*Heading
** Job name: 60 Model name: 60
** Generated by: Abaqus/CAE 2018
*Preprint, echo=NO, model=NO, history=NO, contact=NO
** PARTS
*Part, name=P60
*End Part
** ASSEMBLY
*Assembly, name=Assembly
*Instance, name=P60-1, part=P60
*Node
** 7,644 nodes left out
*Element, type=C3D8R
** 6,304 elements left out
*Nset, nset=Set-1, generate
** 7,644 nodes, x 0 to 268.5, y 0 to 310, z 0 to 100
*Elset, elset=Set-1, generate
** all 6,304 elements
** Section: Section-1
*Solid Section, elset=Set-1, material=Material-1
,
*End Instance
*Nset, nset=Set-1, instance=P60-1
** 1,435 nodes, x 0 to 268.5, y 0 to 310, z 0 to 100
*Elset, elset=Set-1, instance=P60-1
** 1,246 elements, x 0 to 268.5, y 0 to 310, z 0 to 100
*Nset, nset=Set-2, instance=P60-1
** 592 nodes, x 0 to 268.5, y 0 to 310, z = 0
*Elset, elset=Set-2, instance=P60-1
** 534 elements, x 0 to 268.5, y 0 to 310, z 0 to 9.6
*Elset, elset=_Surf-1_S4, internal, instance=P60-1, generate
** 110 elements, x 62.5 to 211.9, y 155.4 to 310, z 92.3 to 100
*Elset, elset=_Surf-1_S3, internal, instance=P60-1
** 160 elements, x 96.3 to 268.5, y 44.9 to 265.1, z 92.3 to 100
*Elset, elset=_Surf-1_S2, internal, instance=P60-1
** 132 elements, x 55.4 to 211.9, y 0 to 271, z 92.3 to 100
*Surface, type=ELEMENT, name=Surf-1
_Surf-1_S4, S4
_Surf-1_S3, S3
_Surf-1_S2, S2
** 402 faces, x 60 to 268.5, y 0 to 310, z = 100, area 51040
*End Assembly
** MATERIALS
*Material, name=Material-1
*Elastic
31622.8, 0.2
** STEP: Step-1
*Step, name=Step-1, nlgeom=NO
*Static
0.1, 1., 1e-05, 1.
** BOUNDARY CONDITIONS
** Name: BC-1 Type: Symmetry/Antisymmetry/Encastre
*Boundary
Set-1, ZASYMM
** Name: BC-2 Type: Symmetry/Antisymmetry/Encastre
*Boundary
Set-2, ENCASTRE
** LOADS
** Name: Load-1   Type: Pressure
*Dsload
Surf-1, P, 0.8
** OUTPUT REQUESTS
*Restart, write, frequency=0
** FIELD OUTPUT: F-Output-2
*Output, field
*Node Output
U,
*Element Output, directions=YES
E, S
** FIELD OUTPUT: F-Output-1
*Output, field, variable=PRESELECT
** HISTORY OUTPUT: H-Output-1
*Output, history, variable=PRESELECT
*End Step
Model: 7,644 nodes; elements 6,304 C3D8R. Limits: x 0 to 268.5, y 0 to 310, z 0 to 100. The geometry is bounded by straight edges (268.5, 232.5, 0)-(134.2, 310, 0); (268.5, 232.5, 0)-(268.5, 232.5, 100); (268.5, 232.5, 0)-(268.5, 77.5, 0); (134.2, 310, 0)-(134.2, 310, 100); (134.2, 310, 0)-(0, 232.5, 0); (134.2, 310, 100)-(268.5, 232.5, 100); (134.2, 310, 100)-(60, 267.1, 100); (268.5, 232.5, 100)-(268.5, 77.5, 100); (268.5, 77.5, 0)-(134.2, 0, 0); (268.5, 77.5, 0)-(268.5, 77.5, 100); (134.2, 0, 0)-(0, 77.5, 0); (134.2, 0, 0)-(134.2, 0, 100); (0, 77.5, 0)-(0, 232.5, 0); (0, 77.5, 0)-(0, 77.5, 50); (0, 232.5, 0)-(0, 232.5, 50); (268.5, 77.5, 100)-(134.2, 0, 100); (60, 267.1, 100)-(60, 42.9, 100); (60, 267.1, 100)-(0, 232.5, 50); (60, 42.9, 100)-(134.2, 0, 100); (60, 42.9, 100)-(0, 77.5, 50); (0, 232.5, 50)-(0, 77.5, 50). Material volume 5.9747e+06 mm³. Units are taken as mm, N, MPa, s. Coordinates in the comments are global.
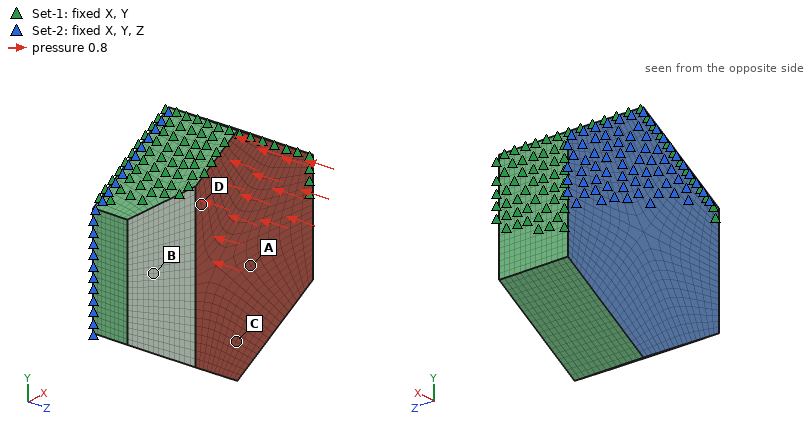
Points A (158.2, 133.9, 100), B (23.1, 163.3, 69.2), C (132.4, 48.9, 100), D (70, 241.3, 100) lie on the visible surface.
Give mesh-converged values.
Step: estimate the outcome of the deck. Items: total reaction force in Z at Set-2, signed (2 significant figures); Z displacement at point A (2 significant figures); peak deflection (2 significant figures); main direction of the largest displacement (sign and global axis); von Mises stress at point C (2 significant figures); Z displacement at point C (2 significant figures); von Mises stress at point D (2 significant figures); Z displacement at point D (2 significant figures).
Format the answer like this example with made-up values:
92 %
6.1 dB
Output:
41000 N
-0.0023 mm
0.0023 mm
-Z
0.57 MPa
-0.0022 mm
0.51 MPa
-0.0017 mm
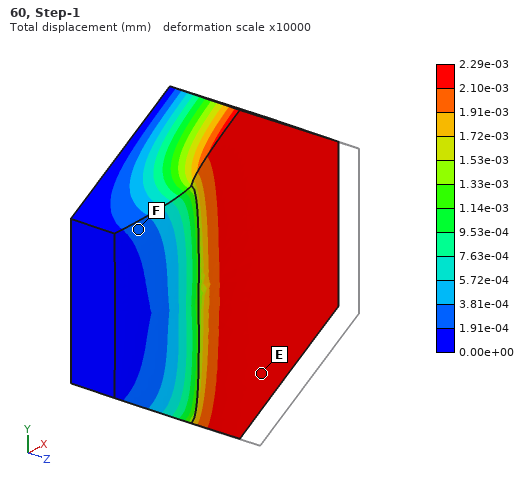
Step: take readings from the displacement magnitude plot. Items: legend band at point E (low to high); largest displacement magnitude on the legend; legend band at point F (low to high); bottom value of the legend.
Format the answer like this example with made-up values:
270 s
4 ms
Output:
2.10e-03 to 2.29e-03 mm
2.29e-03 mm
1.91e-04 to 3.81e-04 mm
0.00e+00 mm
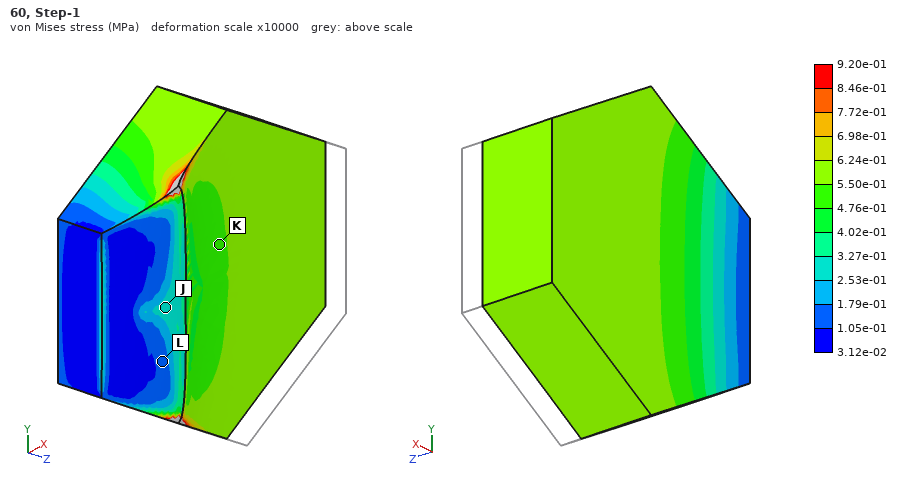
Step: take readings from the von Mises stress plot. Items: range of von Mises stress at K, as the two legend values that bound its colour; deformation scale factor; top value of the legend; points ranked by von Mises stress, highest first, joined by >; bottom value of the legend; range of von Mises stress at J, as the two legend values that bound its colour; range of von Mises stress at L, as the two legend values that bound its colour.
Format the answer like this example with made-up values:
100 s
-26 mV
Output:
4.76e-01 to 5.50e-01 MPa
10000
9.20e-01 MPa
K > J > L
3.12e-02 MPa
2.53e-01 to 3.27e-01 MPa
1.05e-01 to 1.79e-01 MPa
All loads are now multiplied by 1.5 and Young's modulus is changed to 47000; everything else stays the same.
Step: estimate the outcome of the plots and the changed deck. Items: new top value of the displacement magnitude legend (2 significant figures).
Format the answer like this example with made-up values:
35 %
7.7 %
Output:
0.0023 mm
